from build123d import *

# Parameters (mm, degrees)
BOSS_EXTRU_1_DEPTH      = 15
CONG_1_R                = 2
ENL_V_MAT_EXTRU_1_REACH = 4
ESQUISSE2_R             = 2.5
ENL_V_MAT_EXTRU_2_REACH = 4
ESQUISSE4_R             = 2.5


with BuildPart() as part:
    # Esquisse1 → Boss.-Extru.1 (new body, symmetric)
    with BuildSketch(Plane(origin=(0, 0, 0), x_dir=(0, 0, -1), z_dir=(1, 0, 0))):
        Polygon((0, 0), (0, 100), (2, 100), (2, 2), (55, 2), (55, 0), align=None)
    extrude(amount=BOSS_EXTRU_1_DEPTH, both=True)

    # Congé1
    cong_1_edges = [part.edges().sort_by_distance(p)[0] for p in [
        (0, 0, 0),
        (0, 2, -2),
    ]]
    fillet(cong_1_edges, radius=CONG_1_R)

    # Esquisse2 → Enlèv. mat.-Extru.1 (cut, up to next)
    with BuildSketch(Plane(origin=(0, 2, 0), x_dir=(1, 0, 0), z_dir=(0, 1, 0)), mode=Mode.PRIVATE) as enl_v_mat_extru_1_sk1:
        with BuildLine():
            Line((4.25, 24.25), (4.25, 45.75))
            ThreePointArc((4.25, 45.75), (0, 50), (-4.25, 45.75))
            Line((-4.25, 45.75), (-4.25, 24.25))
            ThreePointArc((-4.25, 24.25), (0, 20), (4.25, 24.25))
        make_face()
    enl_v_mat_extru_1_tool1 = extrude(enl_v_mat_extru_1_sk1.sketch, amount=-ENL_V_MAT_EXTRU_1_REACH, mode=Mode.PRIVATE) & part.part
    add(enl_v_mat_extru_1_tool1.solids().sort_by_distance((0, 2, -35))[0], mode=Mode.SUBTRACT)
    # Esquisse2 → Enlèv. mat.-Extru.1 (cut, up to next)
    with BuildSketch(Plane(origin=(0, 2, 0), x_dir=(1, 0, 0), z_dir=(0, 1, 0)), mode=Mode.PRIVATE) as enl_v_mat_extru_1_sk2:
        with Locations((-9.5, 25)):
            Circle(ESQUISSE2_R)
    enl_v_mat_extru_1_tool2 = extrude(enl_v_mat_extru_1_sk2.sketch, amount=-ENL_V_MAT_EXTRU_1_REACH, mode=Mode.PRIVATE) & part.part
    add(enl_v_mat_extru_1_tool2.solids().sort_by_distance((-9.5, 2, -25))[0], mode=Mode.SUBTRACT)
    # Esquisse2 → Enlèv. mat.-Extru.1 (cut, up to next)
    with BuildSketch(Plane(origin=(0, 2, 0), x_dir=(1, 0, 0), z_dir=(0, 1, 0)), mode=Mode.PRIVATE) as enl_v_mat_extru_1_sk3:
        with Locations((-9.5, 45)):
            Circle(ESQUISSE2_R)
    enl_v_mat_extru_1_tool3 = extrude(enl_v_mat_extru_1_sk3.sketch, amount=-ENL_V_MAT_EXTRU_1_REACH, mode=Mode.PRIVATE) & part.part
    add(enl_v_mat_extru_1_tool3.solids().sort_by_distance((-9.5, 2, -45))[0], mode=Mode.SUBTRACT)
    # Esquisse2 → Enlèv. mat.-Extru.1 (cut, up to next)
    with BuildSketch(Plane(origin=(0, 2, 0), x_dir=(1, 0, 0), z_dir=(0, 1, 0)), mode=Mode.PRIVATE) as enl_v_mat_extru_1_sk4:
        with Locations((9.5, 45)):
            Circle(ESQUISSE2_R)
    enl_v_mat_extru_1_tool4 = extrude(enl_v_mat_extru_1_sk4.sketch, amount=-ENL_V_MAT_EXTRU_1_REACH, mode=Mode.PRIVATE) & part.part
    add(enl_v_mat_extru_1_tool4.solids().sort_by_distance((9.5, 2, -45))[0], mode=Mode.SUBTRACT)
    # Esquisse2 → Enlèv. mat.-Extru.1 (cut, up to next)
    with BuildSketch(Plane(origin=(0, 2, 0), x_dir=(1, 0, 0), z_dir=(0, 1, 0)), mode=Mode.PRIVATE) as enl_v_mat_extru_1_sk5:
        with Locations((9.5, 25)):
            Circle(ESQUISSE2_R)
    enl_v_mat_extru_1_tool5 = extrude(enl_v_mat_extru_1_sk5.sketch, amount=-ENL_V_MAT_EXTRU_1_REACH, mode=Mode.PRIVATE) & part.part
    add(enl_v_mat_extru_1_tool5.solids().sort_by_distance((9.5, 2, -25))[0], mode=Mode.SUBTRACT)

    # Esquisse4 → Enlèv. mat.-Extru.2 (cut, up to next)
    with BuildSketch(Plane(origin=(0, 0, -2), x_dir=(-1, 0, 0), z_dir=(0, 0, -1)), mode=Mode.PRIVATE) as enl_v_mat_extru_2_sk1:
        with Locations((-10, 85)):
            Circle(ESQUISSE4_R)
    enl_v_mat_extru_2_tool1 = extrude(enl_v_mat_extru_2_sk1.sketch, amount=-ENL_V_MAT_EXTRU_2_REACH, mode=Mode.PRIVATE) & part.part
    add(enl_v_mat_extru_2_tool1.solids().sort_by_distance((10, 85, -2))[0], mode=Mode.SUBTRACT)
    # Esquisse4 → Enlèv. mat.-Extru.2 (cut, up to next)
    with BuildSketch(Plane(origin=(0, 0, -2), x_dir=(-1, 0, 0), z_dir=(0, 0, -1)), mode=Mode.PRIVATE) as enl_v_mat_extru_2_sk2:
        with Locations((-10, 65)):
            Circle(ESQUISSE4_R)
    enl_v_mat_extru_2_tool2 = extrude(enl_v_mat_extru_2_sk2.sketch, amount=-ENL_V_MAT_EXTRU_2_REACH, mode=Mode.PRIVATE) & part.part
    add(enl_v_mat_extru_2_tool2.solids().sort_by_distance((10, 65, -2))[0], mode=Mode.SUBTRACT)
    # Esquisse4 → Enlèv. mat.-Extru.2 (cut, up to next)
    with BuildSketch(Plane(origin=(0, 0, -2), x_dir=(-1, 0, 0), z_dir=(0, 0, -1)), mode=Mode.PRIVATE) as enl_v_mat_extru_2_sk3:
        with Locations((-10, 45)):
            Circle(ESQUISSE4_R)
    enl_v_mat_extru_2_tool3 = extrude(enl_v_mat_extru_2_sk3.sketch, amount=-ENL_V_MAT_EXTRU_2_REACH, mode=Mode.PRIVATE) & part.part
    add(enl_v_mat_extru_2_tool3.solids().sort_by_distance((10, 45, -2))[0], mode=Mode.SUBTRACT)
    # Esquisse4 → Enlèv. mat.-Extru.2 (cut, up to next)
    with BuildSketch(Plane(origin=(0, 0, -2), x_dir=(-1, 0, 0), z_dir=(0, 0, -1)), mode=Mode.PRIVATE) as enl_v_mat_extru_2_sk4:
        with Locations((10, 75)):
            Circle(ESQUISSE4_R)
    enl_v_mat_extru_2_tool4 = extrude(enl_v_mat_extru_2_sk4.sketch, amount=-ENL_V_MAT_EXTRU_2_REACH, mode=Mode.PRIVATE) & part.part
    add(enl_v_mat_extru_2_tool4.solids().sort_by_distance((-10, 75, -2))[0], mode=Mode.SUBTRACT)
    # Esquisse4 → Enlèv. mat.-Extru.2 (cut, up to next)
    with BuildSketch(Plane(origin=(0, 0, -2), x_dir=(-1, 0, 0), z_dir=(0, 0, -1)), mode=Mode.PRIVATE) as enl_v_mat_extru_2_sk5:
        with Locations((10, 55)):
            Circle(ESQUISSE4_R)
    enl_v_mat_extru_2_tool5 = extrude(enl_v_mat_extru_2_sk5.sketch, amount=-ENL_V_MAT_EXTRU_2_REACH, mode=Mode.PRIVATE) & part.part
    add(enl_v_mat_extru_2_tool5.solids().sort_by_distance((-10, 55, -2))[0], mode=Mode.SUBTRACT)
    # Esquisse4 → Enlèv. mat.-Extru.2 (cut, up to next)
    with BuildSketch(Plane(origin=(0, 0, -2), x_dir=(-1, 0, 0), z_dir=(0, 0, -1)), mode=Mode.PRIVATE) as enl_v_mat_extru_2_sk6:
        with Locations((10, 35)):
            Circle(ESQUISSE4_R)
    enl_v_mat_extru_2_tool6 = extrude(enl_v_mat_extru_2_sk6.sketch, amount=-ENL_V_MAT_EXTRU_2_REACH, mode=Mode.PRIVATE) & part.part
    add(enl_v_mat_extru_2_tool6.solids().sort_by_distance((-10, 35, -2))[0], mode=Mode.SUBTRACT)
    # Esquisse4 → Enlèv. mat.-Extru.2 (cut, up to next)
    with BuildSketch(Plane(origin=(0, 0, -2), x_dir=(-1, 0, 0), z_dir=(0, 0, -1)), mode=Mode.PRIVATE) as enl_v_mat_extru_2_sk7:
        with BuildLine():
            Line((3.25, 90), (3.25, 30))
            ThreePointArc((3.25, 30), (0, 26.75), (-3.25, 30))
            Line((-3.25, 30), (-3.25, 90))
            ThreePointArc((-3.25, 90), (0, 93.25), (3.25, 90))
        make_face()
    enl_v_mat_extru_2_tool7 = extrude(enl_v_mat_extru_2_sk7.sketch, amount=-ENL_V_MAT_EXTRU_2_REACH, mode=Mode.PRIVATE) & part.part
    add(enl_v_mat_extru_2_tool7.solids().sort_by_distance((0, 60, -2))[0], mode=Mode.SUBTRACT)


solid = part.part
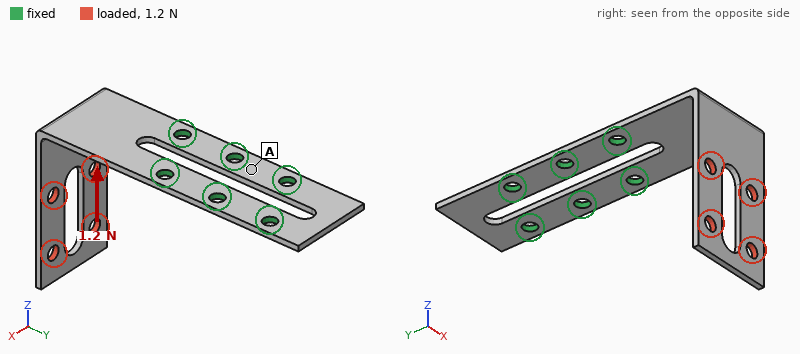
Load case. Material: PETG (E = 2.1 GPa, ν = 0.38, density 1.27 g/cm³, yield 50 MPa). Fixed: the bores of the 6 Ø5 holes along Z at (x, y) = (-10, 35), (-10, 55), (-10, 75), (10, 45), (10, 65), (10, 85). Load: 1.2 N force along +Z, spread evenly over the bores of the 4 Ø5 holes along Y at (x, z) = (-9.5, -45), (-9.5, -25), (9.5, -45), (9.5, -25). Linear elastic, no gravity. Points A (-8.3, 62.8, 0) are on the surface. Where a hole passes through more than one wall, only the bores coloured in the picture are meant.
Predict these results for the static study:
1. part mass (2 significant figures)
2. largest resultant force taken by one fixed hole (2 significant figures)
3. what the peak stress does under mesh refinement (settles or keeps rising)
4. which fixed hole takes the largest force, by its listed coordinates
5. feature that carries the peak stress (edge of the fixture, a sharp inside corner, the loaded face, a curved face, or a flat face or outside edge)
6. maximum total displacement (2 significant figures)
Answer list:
9.5 g
1.3 N
keeps rising
(-10, 35)
edge of the fixture
1.2 mm
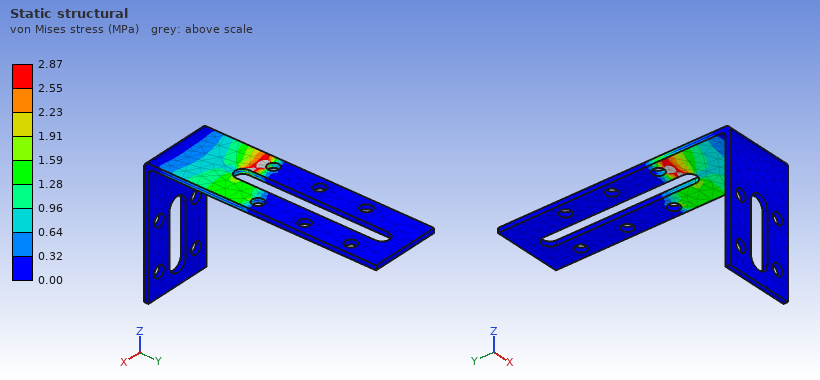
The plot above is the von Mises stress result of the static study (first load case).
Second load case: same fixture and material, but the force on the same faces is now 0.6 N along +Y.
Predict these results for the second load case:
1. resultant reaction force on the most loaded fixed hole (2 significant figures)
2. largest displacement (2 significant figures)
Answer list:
0.44 N
1.3 mm
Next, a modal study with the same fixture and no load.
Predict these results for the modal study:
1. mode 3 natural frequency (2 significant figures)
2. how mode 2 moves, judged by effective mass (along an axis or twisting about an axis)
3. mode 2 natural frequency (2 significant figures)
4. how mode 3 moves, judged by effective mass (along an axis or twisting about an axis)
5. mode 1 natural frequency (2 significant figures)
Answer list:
220 Hz
along X
130 Hz
along Z
76 Hz
